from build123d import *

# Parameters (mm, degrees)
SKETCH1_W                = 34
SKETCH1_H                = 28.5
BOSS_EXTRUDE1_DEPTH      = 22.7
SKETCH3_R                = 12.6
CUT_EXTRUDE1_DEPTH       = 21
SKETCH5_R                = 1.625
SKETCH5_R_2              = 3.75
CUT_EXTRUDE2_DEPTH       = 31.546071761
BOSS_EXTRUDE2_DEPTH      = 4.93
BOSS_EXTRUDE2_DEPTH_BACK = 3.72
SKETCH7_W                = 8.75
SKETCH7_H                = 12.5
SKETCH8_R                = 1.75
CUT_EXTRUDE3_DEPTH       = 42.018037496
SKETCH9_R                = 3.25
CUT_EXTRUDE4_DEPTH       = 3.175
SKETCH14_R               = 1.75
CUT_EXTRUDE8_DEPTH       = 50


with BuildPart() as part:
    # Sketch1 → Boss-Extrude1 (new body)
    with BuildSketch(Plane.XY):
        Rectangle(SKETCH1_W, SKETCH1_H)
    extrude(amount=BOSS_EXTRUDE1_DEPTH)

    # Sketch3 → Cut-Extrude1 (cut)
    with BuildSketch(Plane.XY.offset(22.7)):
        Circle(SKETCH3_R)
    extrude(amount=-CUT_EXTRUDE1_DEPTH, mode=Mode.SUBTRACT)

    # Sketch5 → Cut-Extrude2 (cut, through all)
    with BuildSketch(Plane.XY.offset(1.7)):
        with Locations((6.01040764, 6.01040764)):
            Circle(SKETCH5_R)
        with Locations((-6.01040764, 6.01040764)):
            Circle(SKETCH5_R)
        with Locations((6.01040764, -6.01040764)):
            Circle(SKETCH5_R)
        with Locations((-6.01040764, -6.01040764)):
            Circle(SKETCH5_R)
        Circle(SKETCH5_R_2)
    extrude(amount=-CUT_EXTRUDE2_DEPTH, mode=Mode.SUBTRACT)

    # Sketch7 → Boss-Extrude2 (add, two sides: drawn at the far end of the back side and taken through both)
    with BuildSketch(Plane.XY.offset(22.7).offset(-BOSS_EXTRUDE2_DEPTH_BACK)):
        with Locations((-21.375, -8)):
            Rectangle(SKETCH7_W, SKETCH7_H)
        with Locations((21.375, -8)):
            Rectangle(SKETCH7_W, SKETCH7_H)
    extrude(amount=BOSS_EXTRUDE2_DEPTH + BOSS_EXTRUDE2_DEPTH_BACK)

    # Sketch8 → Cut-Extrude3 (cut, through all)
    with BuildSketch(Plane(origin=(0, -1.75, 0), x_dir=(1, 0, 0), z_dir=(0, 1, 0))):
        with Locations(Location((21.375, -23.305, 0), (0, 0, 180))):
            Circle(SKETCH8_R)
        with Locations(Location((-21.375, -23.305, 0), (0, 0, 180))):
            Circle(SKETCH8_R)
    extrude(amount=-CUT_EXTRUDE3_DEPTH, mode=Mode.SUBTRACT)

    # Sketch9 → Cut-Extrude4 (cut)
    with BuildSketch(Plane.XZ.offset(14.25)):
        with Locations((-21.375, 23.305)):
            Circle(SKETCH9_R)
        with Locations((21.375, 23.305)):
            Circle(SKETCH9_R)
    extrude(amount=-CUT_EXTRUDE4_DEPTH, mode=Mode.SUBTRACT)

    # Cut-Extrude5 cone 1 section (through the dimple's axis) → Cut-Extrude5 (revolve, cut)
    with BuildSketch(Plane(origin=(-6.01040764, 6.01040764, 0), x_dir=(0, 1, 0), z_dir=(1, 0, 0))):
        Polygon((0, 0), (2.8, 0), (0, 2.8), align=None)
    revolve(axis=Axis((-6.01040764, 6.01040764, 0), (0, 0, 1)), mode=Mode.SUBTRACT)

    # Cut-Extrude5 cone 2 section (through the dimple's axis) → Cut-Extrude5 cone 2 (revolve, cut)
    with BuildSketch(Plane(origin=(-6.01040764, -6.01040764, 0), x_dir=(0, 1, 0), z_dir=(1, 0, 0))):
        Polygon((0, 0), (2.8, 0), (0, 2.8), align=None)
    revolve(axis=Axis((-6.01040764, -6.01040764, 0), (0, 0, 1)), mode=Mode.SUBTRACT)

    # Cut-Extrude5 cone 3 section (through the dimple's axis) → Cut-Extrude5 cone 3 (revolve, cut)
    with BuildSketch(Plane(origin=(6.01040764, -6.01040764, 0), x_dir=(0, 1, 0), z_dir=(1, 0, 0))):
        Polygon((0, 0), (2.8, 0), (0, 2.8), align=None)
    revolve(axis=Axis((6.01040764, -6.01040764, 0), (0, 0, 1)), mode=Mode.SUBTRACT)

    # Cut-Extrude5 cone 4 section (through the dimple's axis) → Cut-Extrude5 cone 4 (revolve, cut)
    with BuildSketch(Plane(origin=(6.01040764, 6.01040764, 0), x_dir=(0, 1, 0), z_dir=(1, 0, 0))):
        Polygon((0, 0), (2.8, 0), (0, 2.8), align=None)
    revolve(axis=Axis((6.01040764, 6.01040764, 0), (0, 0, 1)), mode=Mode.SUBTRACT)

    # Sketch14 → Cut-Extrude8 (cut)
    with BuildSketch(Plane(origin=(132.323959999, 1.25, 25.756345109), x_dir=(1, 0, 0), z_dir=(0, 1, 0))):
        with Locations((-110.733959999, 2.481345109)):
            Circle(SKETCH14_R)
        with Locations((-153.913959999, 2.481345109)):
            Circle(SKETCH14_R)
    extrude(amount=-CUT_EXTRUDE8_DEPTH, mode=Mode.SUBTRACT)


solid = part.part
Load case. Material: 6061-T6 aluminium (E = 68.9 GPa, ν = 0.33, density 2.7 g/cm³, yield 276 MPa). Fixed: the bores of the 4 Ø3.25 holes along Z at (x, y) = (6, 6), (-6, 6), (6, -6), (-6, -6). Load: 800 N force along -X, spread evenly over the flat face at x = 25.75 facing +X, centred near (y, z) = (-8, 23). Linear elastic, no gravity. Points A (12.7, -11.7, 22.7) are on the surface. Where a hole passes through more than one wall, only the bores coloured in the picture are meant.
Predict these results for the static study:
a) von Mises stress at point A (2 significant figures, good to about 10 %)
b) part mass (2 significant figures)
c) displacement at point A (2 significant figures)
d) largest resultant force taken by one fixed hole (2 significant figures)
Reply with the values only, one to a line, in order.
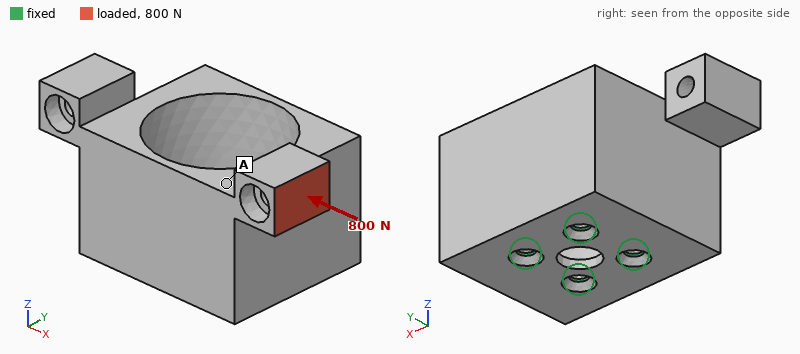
50 MPa
35 g
0.12 mm
710 N
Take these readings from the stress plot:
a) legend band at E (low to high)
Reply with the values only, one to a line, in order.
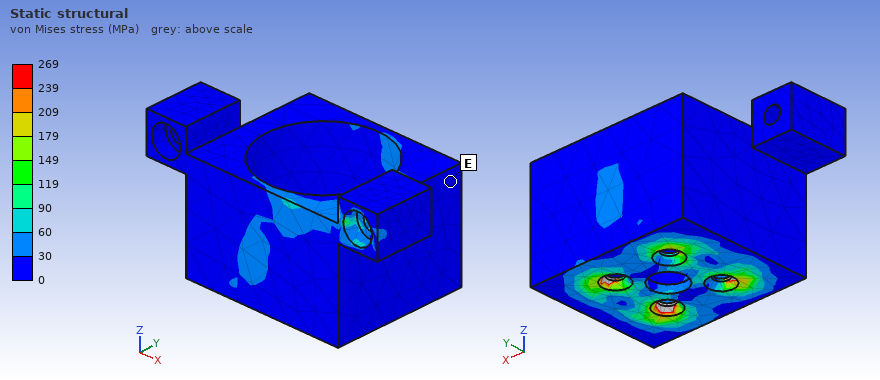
0 to 30 MPa
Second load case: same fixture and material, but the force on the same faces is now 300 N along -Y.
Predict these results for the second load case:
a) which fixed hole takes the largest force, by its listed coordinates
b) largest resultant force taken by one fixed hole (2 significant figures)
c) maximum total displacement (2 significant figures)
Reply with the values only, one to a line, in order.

(6, 6)
370 N
68 µm
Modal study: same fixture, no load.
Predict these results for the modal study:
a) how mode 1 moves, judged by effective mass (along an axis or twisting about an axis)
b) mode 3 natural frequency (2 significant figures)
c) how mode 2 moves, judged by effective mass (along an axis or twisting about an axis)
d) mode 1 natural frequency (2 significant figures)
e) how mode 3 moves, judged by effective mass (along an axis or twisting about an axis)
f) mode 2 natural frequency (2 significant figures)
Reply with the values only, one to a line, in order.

along X
7600 Hz
along Y
2900 Hz
along Z
3400 Hz
